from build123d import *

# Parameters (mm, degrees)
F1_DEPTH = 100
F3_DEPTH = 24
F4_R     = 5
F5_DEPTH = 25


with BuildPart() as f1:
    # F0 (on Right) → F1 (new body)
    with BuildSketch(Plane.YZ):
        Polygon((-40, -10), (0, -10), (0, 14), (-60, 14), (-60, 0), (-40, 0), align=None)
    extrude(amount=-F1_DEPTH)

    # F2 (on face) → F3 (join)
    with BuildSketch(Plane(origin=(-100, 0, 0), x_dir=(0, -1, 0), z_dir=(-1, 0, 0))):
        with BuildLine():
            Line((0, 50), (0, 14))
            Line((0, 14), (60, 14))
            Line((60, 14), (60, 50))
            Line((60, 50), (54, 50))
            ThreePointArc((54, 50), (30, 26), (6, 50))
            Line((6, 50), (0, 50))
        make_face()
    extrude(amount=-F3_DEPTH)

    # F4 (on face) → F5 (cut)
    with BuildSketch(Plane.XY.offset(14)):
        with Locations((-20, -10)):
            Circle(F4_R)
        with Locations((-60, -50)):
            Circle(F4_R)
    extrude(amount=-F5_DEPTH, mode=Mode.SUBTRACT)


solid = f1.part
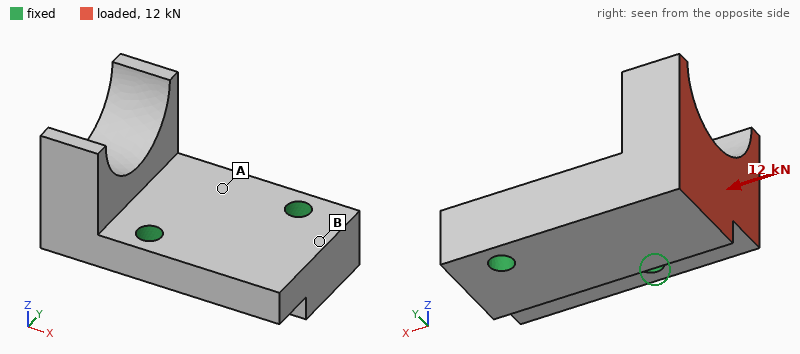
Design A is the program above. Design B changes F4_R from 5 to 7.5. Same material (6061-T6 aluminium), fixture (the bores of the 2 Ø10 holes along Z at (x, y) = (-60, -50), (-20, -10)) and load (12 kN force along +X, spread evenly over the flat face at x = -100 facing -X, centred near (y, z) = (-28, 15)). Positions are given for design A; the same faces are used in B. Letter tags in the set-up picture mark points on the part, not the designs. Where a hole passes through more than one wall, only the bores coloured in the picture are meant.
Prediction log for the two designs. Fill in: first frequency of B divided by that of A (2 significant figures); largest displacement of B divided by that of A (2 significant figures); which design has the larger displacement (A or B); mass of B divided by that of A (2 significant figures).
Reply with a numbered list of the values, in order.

1. 1.1
2. 0.88
3. A
4. 0.98
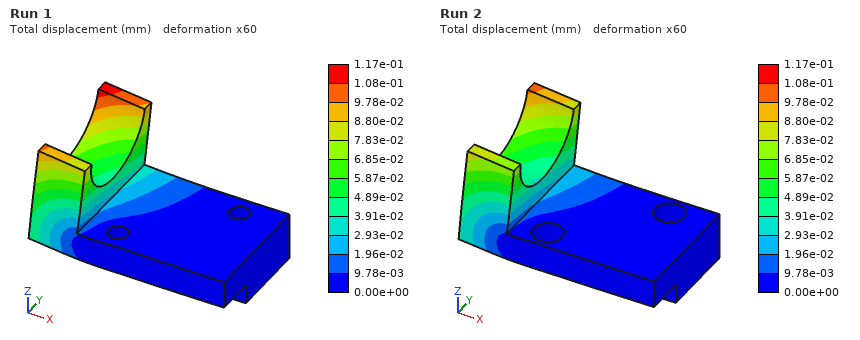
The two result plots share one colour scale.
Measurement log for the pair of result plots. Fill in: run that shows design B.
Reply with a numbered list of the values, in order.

1. Run 2
